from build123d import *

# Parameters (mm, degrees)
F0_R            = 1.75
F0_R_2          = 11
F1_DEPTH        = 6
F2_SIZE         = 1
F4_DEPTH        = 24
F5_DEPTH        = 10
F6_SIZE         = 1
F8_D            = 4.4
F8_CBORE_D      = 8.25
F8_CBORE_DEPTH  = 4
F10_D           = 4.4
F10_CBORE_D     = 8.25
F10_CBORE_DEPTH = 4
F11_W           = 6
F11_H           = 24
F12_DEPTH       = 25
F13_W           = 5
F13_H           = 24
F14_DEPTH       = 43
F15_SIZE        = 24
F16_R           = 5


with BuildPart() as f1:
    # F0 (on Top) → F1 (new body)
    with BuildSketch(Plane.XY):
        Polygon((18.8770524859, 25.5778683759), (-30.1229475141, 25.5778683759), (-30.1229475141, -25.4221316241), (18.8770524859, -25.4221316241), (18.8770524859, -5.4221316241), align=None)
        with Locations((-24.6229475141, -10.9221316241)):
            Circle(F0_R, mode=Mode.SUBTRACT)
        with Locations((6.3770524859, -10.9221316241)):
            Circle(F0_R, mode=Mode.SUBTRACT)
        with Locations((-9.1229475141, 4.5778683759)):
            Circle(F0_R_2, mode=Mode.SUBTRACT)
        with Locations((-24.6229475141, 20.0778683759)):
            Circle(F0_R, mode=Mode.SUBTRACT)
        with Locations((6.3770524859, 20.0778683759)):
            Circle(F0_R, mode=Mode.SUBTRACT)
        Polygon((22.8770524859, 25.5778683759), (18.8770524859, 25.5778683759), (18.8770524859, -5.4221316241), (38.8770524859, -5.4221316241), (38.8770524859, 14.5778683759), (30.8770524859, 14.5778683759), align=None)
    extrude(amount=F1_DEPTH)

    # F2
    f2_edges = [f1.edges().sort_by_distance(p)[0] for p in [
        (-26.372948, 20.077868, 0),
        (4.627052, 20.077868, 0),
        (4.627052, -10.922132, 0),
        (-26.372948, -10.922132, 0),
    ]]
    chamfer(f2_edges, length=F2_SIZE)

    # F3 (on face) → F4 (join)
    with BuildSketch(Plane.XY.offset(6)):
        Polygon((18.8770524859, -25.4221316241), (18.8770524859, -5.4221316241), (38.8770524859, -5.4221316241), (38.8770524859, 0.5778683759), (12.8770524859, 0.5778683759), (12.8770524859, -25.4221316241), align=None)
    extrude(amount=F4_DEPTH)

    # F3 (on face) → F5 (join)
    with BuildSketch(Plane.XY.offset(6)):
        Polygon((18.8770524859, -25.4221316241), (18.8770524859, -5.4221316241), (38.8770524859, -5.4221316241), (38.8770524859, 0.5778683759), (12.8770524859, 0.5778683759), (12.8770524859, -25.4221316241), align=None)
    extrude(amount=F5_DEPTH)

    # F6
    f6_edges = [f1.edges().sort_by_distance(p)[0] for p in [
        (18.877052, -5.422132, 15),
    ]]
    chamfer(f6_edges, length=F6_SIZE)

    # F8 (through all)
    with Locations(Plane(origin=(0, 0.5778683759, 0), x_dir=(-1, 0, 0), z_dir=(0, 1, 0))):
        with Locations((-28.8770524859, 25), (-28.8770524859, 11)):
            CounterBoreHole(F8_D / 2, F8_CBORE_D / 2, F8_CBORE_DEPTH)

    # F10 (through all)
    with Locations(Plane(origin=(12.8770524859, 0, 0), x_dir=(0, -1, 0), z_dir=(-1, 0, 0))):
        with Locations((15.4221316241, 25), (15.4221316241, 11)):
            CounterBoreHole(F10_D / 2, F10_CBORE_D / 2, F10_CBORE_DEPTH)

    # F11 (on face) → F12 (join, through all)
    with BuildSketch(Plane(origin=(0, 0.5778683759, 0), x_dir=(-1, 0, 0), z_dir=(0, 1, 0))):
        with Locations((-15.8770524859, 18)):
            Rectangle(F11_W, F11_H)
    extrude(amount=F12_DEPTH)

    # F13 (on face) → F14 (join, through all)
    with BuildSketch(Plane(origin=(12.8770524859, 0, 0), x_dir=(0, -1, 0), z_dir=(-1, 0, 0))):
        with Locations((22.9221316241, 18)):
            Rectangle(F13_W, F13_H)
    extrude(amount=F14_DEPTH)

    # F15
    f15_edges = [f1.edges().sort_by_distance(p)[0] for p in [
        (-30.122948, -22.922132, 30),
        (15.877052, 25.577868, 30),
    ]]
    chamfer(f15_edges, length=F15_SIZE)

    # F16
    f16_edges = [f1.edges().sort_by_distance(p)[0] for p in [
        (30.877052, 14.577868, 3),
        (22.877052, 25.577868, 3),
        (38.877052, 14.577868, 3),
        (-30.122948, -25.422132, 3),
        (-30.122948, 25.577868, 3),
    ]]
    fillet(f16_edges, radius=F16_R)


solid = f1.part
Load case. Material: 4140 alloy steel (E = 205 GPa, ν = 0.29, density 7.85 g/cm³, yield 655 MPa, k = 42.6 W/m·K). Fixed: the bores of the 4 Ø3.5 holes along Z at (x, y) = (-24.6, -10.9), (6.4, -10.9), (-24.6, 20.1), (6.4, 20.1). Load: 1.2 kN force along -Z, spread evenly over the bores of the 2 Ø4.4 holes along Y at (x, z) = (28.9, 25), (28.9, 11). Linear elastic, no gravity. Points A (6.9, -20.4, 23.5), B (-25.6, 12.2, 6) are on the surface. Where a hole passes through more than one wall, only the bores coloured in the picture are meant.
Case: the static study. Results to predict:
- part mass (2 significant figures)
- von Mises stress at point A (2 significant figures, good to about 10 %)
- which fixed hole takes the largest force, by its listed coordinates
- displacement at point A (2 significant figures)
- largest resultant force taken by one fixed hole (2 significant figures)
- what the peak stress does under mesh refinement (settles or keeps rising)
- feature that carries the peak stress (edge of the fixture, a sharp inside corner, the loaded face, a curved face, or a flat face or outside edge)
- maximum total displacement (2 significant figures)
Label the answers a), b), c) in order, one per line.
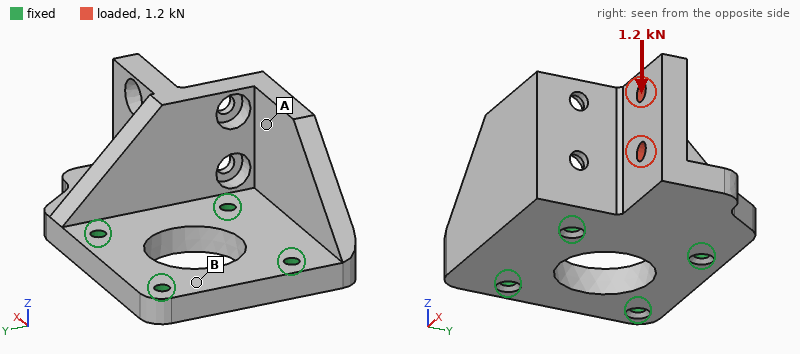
a) 210 g
b) 22 MPa
c) (6.4, -10.9)
d) 8.7 µm
e) 1.4 kN
f) keeps rising
g) edge of the fixture
h) 44 µm
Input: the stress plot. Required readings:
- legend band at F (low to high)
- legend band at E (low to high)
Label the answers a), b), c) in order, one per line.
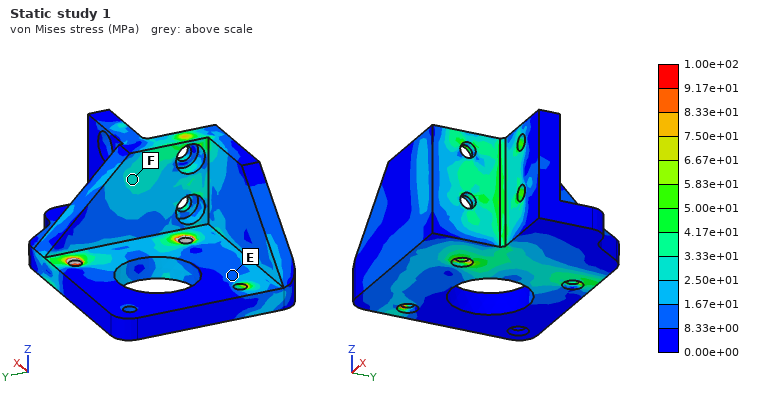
a) 2.50e+01 to 3.33e+01 MPa
b) 8.33e+00 to 1.67e+01 MPa
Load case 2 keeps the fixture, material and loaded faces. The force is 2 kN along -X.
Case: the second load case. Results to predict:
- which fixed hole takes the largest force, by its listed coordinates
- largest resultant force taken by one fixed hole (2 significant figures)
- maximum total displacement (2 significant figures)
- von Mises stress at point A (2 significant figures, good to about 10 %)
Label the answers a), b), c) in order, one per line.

a) (6.4, -10.9)
b) 1.4 kN
c) 54 µm
d) 34 MPa
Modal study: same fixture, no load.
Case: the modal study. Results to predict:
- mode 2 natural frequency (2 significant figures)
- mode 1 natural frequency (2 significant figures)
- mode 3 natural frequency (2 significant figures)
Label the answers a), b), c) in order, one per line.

a) 7200 Hz
b) 4300 Hz
c) 11 kHz
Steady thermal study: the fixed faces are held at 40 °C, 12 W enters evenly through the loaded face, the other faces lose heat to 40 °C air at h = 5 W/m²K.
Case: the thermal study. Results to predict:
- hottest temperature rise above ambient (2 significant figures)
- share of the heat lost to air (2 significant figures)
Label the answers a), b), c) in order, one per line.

a) 52 K
b) 5.4 %
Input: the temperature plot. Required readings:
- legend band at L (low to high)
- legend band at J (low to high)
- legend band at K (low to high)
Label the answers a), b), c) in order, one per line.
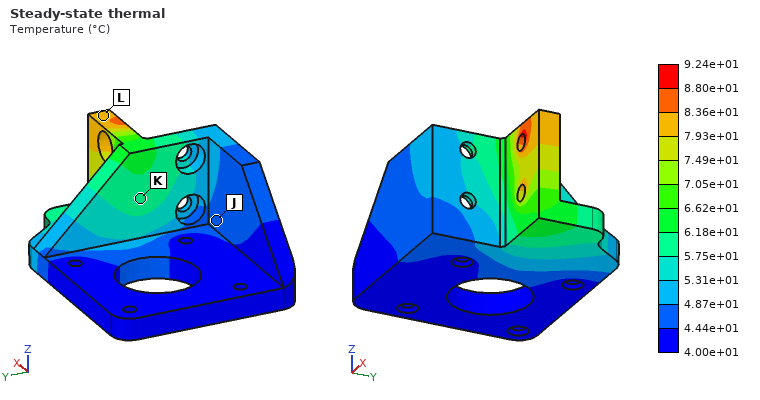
a) 7.93e+01 to 8.36e+01 °C
b) 4.44e+01 to 4.87e+01 °C
c) 5.75e+01 to 6.18e+01 °C
